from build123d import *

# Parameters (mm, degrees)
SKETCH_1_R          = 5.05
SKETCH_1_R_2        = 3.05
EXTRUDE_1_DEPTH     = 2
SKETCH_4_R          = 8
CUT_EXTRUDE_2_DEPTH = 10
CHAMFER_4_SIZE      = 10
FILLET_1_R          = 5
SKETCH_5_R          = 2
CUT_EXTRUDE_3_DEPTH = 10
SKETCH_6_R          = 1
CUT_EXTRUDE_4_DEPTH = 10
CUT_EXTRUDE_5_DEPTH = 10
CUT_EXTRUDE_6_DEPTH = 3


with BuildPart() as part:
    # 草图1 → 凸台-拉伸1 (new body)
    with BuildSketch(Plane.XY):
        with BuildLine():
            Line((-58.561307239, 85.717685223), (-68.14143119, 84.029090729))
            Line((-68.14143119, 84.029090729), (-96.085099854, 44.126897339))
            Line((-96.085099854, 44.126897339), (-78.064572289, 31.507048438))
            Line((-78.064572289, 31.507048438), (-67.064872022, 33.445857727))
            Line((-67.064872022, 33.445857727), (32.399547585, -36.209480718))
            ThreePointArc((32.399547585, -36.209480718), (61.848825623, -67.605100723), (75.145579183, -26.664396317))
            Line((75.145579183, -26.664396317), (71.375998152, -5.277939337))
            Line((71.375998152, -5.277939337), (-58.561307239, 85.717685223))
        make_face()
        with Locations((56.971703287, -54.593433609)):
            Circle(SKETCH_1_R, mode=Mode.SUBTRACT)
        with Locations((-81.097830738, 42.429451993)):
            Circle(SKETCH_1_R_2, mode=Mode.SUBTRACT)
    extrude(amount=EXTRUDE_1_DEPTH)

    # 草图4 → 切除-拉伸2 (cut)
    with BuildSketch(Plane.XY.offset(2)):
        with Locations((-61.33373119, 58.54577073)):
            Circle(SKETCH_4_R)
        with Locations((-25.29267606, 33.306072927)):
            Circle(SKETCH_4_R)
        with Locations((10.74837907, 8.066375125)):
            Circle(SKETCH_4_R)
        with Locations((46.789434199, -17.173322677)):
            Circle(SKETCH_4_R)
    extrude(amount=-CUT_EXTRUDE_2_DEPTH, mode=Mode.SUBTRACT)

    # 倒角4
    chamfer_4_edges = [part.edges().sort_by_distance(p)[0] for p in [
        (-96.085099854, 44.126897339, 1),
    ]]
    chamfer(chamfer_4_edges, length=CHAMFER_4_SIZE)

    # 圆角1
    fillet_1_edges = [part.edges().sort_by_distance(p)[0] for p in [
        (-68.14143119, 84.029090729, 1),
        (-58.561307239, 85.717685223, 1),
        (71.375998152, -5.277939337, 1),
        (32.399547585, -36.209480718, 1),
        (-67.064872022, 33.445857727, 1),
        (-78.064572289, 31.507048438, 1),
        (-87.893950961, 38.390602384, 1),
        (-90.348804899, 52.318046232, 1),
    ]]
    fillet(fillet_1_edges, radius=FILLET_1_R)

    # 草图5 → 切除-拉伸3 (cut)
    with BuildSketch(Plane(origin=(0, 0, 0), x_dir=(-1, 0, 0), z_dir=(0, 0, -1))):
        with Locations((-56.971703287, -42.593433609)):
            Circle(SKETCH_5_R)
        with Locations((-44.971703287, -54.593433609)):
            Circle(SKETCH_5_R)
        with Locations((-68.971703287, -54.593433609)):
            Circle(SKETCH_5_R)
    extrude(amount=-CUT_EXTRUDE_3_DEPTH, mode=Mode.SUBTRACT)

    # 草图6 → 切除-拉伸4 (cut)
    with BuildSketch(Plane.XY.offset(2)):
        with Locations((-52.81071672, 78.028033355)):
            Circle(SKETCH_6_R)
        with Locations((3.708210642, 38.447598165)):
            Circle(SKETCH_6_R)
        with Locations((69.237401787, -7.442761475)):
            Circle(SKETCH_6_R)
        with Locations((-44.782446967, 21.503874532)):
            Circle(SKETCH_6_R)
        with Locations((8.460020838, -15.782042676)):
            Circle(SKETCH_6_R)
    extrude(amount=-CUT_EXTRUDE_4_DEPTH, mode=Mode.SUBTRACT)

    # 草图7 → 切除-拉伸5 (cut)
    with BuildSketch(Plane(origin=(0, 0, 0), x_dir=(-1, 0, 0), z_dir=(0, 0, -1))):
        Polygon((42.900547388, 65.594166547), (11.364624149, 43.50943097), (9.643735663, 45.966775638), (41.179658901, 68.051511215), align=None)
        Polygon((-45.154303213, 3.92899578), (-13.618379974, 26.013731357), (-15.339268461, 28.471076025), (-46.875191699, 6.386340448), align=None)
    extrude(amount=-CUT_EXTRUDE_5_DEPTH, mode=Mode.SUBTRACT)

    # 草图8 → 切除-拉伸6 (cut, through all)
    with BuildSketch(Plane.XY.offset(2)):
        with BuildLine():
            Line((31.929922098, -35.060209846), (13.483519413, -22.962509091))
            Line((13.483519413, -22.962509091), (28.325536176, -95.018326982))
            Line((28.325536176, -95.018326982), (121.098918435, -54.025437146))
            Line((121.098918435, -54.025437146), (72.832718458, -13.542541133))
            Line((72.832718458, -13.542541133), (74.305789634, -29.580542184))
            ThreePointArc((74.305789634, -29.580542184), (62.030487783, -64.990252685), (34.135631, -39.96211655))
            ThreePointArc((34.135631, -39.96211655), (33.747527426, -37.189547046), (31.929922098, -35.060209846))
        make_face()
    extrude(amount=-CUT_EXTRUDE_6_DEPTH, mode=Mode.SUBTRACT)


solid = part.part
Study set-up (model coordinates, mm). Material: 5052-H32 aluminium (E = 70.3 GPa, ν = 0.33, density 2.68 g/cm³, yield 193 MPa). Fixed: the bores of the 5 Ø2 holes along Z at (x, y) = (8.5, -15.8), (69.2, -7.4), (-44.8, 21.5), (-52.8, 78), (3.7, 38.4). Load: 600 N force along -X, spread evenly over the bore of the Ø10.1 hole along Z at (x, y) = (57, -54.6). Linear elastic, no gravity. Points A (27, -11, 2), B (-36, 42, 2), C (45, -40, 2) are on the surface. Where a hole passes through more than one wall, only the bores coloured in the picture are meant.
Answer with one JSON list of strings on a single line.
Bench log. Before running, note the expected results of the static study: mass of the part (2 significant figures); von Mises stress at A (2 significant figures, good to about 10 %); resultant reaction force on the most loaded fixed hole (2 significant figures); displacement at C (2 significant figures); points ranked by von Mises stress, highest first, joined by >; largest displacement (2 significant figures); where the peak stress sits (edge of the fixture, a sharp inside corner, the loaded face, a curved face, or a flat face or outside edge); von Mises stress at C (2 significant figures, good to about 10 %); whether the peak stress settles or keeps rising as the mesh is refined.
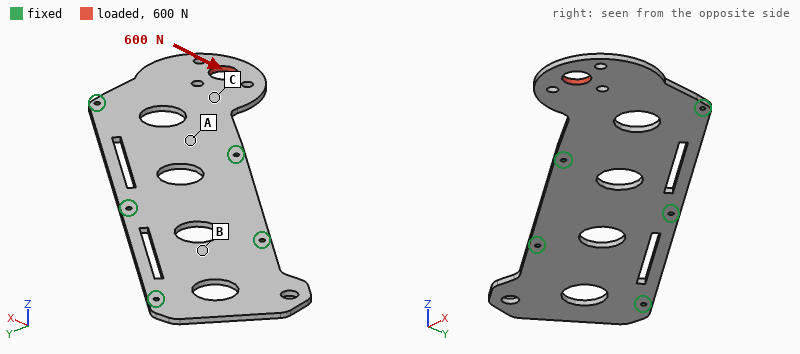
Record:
["44 g", "7.8 MPa", "490 N", "17 µm", "C > A > B", "41 µm", "edge of the fixture", "19 MPa", "keeps rising"]
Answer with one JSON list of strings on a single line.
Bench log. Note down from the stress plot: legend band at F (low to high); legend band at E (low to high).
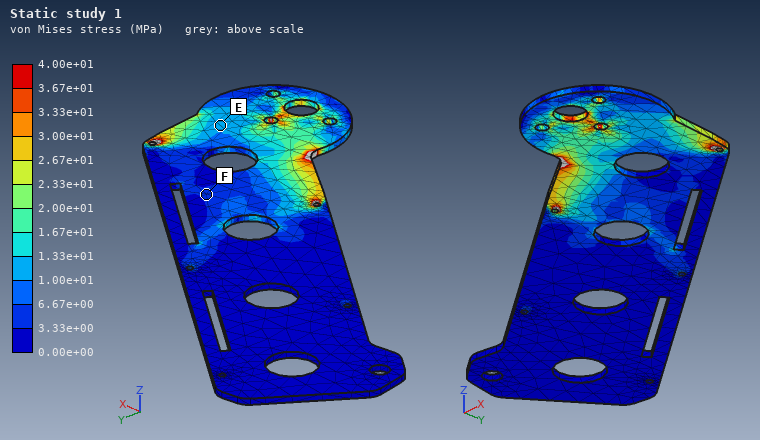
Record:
["3.33e+00 to 6.67e+00 MPa", "1.00e+01 to 1.33e+01 MPa"]
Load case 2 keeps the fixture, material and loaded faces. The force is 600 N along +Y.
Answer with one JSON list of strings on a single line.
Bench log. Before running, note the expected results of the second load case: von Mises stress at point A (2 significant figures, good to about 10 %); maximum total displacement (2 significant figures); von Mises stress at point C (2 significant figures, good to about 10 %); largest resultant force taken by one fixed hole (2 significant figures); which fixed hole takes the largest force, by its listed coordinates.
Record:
["3.6 MPa", "12 µm", "6.2 MPa", "440 N", "(69.2, -7.4)"]
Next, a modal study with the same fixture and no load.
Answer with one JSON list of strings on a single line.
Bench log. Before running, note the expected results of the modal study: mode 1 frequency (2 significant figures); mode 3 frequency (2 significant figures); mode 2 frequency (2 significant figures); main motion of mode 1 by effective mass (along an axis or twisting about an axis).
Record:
["510 Hz", "1700 Hz", "1000 Hz", "along Z"]
